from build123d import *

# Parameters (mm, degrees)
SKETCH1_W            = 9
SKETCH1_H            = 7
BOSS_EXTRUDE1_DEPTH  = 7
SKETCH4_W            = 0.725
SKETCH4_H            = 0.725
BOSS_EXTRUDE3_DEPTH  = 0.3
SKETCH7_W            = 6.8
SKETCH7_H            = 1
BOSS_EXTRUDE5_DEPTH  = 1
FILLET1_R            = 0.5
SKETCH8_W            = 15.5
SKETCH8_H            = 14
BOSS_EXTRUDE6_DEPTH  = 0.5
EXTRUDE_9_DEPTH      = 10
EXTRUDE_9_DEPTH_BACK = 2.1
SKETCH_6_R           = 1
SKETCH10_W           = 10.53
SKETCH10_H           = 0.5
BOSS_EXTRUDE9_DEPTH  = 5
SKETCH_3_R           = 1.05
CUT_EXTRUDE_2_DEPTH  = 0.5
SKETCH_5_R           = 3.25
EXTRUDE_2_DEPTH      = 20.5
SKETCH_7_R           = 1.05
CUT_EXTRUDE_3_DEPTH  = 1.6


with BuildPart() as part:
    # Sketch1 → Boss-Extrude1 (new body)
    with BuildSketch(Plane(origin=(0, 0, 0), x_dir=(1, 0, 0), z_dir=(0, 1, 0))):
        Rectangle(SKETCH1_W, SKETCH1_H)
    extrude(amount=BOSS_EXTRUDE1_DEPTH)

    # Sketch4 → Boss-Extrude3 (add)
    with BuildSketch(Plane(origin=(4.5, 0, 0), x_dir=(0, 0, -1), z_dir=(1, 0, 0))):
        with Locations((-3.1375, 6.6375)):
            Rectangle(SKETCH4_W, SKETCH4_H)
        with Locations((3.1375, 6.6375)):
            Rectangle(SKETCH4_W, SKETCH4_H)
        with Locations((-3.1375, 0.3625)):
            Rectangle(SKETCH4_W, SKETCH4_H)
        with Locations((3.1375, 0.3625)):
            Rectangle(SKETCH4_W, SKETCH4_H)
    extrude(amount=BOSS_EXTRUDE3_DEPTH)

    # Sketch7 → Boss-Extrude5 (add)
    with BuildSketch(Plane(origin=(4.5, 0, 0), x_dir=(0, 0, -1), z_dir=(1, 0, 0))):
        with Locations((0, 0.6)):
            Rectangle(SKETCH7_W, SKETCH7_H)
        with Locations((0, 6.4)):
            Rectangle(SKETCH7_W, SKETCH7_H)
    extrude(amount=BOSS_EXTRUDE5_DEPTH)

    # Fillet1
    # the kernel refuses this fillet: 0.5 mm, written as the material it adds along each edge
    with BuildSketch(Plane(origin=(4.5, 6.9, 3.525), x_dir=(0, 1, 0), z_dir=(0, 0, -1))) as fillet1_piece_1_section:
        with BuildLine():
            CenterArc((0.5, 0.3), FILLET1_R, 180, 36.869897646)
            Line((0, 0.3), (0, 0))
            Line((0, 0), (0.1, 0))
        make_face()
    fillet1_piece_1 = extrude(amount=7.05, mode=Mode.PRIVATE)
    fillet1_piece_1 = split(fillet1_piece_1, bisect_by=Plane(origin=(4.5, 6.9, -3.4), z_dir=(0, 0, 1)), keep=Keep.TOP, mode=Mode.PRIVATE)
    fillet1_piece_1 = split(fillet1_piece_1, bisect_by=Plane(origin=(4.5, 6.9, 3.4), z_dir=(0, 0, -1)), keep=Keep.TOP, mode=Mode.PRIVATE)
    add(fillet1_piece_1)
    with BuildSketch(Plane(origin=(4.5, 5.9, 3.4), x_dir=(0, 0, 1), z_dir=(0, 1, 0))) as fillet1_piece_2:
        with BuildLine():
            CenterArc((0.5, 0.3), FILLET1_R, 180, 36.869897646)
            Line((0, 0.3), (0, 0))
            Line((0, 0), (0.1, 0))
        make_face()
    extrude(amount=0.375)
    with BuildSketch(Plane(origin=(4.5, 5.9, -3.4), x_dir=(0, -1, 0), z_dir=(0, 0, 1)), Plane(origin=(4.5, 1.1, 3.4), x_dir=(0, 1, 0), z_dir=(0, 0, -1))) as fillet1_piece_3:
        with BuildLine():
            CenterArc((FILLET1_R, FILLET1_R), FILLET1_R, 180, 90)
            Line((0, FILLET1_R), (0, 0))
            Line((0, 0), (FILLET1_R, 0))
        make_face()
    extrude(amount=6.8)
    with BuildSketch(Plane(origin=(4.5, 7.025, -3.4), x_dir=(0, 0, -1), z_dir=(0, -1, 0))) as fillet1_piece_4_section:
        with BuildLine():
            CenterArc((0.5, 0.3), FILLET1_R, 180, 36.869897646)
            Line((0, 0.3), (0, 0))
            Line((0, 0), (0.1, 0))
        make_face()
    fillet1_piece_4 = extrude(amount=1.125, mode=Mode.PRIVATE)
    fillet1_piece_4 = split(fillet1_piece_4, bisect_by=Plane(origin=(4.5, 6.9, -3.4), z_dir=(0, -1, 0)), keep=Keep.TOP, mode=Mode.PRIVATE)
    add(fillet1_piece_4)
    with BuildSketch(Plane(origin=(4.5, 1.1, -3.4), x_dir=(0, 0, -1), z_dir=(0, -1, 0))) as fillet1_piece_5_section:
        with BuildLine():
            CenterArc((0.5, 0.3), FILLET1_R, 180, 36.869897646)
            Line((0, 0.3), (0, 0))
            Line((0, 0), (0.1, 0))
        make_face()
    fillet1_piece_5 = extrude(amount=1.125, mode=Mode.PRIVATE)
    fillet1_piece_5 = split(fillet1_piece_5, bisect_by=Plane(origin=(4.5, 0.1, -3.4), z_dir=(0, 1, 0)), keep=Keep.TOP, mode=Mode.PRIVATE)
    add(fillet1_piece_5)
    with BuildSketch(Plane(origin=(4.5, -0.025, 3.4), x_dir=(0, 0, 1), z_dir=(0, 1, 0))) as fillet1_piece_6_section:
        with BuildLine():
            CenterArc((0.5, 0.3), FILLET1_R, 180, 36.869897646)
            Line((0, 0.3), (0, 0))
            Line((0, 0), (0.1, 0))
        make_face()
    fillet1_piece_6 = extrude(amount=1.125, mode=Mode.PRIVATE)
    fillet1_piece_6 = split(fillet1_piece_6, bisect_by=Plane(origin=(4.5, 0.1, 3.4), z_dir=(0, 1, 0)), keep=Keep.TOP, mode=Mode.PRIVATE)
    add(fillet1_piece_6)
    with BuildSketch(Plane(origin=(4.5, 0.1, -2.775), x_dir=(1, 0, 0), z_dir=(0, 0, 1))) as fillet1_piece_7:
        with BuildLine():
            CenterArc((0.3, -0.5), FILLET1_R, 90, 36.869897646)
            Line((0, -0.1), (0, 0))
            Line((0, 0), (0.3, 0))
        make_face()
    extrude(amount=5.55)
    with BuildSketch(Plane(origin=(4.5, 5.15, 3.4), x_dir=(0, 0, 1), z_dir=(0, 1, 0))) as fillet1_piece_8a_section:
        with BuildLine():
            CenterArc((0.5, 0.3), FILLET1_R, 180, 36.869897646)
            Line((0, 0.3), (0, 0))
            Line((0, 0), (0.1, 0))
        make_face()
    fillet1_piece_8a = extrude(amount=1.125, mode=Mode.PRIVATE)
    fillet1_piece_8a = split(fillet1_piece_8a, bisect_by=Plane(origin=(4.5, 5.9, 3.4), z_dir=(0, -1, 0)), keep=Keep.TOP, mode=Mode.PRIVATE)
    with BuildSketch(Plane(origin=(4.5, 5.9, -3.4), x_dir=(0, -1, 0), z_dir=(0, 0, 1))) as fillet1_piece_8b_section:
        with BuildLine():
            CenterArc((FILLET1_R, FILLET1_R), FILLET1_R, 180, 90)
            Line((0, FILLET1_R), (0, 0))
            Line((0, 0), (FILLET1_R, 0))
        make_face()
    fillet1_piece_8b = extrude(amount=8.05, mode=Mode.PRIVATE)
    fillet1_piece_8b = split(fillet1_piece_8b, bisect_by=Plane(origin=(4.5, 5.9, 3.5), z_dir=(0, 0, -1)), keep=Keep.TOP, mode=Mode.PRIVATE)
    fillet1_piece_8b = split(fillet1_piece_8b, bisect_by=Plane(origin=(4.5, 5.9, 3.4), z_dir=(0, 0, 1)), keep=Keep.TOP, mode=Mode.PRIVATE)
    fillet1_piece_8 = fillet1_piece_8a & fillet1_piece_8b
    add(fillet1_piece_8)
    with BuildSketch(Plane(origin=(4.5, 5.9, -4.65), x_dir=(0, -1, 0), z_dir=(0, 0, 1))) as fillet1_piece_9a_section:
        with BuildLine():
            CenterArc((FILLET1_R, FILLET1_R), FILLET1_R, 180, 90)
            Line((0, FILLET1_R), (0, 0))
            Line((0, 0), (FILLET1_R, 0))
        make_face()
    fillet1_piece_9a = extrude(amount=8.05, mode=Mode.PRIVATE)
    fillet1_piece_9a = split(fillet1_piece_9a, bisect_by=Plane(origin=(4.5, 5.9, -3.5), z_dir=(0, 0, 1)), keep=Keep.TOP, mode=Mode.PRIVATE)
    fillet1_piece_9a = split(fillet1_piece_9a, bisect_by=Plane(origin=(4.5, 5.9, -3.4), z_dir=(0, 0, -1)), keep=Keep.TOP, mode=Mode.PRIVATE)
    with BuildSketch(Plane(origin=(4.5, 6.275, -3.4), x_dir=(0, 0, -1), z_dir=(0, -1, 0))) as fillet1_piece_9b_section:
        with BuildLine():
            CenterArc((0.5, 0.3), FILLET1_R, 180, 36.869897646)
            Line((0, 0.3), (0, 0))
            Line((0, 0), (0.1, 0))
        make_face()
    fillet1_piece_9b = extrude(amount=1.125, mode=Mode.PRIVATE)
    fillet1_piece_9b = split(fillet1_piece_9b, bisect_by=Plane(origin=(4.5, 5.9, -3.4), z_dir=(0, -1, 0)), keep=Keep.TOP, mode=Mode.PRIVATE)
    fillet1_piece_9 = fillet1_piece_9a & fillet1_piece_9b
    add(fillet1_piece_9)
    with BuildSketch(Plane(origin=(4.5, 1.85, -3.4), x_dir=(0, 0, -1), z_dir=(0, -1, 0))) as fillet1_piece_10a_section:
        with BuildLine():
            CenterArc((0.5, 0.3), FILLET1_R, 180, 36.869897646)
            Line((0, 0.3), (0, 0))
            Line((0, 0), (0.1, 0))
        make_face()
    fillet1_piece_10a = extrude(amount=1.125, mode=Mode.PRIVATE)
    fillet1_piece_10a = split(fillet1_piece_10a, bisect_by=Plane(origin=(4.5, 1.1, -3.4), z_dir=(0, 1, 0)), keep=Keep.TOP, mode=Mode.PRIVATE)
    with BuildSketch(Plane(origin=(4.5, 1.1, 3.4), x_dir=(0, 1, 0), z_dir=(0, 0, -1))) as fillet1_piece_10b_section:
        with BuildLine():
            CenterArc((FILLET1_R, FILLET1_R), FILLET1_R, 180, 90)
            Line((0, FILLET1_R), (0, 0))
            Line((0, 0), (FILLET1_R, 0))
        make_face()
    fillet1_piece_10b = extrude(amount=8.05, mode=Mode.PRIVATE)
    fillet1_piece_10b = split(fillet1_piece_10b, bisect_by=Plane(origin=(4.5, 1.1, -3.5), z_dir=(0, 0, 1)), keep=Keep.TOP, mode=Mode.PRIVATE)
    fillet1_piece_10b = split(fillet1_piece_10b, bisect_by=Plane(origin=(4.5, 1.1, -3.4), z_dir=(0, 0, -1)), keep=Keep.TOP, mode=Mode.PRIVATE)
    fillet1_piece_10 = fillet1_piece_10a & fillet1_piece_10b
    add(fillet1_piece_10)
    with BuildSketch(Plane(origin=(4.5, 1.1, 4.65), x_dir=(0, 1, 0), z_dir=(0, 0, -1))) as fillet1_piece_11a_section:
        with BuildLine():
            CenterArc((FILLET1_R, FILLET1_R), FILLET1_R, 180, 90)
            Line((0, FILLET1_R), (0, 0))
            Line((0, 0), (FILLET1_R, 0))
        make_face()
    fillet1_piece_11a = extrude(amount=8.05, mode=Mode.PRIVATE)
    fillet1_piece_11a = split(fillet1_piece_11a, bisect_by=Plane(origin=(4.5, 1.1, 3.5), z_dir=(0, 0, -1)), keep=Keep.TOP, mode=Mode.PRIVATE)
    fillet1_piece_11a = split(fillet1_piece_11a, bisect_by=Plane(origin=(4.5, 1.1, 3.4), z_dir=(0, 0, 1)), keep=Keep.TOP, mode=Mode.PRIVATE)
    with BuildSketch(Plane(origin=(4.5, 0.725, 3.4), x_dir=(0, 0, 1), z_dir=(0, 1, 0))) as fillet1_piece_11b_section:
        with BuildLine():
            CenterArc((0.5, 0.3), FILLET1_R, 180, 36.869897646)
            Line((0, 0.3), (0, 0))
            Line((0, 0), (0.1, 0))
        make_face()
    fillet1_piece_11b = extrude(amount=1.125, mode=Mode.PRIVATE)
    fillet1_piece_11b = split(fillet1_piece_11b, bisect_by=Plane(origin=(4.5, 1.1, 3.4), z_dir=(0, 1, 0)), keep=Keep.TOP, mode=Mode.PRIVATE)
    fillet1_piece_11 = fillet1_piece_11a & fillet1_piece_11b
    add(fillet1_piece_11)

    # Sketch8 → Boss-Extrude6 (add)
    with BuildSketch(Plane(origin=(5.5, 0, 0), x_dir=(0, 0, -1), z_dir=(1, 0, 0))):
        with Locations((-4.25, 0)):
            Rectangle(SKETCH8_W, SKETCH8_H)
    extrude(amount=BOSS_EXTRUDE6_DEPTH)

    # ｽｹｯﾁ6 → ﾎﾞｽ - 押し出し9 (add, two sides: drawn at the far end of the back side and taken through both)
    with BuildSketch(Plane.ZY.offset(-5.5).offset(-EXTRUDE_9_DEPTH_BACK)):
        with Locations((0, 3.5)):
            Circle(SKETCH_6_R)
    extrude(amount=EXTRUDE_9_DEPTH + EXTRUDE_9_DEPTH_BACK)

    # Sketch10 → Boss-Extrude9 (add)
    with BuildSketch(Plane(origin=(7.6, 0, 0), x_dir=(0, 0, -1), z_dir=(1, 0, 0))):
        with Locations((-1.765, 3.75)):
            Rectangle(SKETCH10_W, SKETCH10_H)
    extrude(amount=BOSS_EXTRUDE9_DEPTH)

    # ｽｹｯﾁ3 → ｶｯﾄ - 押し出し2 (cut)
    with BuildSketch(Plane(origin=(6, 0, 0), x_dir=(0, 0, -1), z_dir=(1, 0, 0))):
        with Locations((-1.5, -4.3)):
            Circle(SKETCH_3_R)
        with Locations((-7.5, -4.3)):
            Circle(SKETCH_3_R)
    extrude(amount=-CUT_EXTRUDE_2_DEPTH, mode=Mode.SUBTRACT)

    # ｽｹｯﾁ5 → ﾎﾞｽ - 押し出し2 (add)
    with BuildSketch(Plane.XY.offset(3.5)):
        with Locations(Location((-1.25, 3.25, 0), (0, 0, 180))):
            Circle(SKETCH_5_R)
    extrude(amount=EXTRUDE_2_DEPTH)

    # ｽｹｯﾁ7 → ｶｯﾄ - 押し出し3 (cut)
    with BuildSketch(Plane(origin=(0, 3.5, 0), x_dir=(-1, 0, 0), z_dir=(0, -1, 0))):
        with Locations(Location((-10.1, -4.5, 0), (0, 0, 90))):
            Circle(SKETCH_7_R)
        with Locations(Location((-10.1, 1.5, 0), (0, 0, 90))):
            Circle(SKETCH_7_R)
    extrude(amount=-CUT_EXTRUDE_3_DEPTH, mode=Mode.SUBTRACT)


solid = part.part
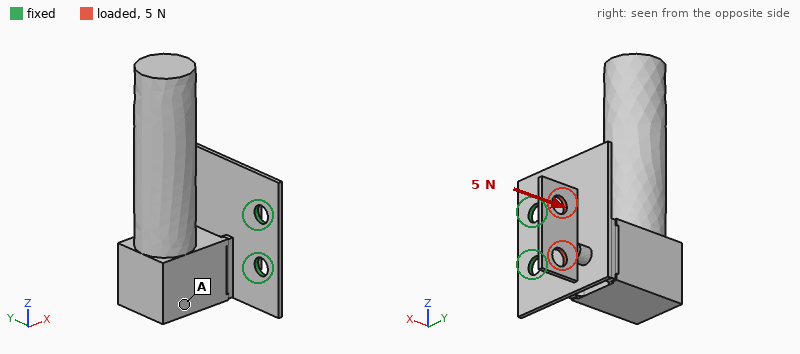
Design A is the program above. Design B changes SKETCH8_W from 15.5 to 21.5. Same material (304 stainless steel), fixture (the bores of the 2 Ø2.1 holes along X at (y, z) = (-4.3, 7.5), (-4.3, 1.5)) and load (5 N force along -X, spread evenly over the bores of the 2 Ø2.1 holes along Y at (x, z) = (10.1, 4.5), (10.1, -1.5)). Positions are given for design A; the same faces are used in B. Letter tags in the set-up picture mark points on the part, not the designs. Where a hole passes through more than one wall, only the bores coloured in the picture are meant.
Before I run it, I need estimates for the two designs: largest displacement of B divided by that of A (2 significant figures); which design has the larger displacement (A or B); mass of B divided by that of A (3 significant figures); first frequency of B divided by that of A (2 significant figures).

0.89
A
1.03
1.1
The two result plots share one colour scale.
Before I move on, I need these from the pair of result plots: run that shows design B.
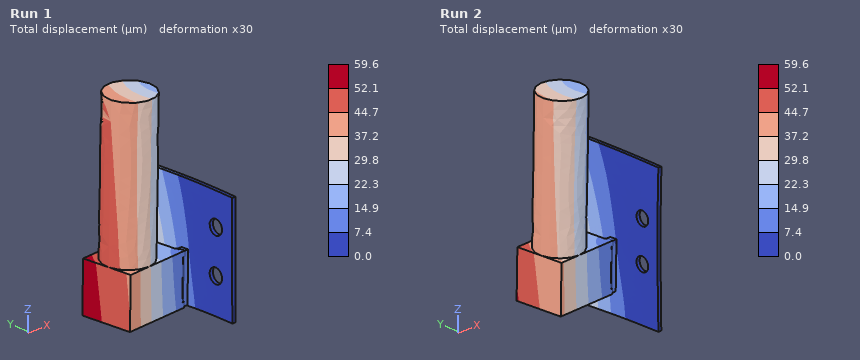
Run 2
